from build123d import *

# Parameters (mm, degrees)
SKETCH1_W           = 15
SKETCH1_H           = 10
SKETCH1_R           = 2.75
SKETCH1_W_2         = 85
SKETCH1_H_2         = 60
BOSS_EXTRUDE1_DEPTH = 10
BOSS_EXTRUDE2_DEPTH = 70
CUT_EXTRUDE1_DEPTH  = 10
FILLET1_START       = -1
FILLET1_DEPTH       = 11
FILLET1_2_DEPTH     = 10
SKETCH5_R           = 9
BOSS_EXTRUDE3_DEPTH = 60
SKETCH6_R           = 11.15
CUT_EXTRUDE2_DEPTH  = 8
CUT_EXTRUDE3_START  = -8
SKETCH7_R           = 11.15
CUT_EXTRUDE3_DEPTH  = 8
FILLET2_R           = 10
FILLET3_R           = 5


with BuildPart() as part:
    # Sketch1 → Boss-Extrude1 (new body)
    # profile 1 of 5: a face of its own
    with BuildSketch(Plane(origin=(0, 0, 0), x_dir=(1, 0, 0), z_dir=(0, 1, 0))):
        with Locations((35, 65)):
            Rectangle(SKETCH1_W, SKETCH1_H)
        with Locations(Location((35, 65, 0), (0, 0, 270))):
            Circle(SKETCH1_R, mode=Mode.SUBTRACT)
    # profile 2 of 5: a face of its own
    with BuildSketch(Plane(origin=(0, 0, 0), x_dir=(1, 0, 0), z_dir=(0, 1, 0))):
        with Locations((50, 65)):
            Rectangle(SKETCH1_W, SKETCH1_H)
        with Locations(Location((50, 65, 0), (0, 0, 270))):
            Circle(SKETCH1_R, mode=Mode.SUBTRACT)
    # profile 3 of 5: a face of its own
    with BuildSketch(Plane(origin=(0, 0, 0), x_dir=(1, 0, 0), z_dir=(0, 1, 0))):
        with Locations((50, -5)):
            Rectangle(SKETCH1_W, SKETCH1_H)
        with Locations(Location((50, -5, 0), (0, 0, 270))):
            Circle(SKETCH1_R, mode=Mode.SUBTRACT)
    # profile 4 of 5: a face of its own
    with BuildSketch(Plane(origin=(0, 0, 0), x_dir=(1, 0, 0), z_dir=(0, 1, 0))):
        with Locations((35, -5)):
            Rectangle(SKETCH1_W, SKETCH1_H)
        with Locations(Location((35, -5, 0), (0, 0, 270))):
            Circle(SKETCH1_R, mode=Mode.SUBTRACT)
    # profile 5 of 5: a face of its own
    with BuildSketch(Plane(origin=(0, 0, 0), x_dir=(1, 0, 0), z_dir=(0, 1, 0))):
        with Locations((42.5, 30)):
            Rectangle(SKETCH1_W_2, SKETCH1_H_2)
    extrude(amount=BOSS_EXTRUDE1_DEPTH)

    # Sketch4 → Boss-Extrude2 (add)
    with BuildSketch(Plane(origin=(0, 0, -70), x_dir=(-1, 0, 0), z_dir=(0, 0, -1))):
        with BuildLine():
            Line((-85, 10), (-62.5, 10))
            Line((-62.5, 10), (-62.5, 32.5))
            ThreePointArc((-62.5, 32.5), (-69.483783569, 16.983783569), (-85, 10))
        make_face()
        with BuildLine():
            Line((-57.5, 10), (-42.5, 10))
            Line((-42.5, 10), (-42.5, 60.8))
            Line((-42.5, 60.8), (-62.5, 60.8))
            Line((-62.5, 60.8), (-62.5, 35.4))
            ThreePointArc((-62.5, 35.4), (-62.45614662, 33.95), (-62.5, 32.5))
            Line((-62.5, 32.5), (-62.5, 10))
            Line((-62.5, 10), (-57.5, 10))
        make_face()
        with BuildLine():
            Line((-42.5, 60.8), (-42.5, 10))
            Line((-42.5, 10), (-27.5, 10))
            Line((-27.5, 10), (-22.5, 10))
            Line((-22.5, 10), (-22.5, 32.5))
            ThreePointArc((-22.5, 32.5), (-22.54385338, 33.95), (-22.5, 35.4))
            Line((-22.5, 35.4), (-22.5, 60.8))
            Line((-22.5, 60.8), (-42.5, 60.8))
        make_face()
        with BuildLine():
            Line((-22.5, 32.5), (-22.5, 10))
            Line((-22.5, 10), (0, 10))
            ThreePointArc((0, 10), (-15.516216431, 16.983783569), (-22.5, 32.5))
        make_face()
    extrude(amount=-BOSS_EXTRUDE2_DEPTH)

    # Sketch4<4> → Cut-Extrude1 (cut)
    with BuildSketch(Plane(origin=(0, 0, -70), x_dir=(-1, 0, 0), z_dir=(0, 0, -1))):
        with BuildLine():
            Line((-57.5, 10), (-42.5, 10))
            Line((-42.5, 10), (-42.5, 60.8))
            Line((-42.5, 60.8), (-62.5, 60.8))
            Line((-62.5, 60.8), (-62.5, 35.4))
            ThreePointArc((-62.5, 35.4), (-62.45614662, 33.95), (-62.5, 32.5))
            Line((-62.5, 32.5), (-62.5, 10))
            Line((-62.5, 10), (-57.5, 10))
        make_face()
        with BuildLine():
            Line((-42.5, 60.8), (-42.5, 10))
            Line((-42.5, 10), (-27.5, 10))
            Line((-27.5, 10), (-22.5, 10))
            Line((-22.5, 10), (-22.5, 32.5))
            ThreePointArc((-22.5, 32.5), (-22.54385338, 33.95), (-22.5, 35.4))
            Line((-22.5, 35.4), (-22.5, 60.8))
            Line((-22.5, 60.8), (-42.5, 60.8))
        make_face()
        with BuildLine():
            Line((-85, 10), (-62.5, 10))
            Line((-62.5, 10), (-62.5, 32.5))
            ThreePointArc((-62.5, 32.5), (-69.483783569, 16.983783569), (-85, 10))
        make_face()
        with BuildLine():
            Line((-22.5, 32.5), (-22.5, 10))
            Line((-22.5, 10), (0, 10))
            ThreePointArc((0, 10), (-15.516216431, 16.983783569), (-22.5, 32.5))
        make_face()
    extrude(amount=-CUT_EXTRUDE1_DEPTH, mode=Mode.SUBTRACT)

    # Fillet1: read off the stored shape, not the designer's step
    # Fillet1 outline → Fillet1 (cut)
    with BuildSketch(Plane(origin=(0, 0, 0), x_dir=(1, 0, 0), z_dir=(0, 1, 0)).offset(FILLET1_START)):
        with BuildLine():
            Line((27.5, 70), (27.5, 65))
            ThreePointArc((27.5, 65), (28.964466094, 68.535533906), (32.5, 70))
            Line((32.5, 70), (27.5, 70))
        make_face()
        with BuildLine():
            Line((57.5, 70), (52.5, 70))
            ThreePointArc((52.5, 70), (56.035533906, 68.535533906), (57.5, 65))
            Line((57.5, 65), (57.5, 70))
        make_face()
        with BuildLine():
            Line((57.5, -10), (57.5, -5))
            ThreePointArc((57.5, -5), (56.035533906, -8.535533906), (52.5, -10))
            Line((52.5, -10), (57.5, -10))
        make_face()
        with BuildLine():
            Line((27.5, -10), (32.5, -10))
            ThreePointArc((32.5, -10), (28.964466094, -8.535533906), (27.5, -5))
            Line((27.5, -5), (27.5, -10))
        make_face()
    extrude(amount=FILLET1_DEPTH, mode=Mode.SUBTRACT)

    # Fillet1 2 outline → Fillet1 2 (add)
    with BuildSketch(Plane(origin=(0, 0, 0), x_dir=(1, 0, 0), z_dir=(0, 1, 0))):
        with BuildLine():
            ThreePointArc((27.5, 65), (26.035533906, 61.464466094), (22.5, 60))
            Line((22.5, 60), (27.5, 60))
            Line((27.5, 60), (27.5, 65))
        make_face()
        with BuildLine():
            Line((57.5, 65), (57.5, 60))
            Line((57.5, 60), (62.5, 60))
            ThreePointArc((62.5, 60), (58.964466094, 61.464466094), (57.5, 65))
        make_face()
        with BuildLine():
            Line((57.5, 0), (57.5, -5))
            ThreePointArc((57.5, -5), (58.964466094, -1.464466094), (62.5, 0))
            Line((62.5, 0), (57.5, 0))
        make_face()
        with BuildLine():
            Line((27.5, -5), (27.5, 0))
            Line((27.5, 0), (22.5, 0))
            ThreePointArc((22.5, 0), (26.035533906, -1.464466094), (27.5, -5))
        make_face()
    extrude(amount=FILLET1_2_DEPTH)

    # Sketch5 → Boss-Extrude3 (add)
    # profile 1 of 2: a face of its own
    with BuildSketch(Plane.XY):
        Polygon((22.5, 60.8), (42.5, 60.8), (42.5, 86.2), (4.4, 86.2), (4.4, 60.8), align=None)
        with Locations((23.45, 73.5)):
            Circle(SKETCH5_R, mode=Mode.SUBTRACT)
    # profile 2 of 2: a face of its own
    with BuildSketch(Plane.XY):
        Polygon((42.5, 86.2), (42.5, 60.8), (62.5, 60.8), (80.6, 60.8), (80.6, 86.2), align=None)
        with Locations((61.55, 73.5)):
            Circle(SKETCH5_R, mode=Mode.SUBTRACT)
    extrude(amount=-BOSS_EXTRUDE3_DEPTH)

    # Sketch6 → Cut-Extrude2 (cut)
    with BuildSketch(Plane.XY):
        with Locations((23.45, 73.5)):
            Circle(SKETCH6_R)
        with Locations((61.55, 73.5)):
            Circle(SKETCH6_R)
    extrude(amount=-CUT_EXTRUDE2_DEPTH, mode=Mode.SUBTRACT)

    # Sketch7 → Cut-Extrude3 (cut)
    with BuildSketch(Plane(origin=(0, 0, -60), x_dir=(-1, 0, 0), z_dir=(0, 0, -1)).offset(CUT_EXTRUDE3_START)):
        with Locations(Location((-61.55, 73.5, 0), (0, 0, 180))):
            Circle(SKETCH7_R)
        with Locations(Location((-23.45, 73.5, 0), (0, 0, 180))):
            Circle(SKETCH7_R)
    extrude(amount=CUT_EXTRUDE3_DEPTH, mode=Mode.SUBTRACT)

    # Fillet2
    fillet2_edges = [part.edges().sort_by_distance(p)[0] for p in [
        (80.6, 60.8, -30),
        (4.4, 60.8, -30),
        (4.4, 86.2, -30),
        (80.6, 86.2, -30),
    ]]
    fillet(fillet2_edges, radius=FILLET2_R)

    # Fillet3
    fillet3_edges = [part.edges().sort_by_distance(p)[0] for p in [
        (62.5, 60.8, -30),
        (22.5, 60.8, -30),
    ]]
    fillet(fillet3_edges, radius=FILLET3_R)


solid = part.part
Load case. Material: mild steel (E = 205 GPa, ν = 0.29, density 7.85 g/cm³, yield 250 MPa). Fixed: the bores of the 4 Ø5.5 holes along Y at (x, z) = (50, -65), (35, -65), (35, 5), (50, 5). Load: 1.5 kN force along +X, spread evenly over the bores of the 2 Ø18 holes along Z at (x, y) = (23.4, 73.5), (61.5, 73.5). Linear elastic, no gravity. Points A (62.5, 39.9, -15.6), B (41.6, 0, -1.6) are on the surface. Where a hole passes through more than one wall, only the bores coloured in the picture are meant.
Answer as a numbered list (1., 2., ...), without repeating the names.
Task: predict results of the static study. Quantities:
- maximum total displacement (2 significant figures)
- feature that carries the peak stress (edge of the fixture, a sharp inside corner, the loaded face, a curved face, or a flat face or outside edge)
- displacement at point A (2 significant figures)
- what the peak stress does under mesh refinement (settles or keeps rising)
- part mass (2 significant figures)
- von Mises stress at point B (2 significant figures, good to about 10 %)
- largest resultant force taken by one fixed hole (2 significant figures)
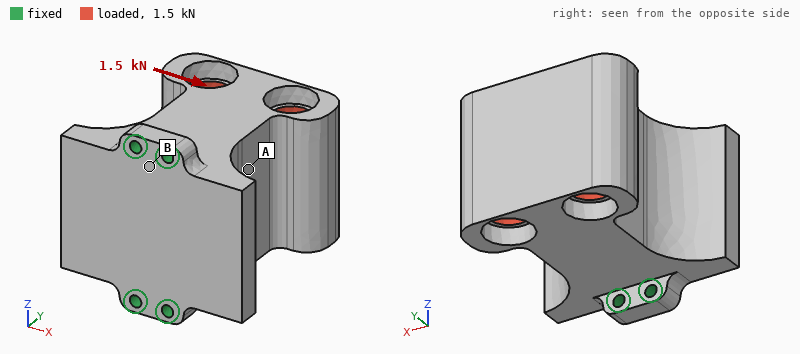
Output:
1. 25 µm
2. edge of the fixture
3. 11 µm
4. keeps rising
5. 2.1 kg
6. 18 MPa
7. 2.3 kN
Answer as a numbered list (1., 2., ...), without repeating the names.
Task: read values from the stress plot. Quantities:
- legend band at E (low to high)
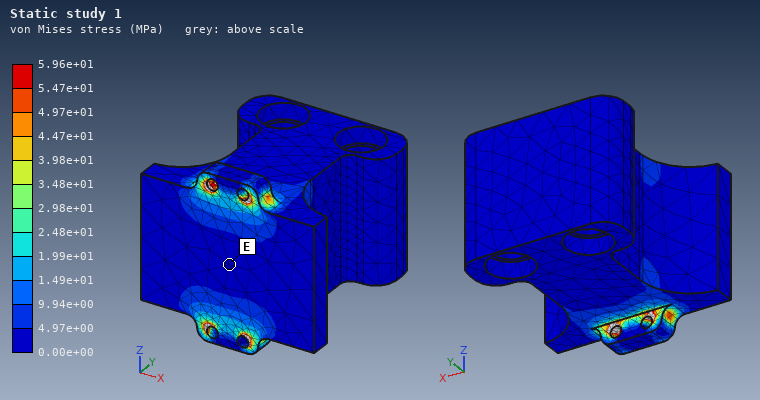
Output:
1. 0.00e+00 to 4.97e+00 MPa
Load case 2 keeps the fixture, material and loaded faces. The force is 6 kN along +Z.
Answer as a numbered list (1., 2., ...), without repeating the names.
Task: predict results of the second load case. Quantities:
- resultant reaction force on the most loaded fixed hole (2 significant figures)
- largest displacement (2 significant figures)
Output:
1. 3.6 kN
2. 16 µm
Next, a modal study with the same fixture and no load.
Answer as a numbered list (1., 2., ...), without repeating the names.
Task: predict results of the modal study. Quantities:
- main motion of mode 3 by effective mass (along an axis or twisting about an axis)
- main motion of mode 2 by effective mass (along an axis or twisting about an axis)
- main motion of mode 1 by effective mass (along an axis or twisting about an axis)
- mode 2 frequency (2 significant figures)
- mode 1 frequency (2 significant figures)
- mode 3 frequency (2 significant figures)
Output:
1. along Y
2. along Z
3. along X
4. 3800 Hz
5. 1400 Hz
6. 6100 Hz
